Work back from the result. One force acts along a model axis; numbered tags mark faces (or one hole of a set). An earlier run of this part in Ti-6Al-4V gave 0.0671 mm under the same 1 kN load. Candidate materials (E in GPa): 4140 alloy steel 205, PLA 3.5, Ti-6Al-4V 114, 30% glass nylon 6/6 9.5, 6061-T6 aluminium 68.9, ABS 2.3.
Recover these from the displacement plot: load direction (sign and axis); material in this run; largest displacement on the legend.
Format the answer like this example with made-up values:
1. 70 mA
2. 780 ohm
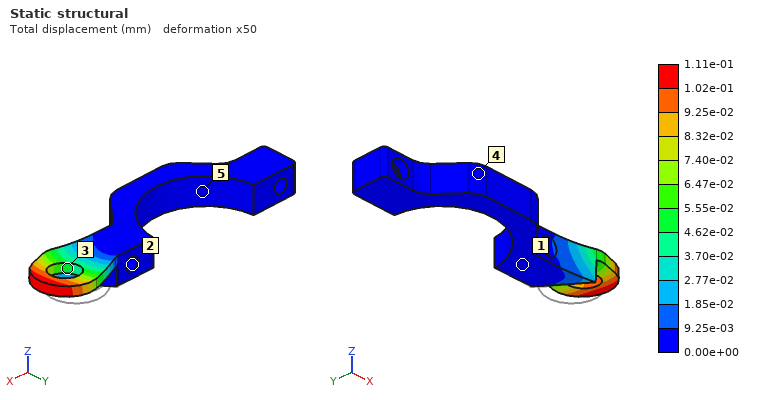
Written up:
1. -Y
2. 6061-T6 aluminium
3. 1.11e-01 mm
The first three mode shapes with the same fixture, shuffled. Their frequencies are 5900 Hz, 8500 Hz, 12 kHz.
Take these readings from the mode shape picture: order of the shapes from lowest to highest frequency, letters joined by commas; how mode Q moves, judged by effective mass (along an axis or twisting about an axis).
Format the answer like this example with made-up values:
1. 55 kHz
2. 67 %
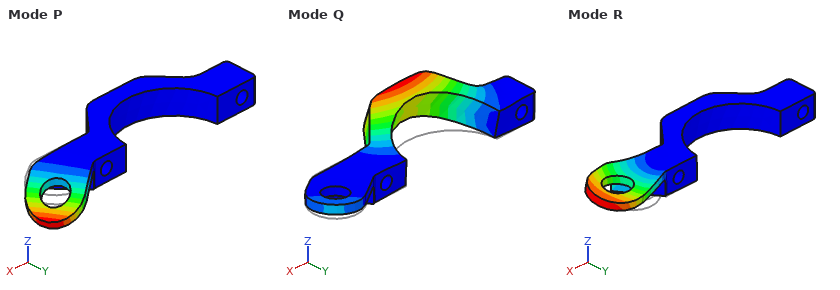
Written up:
1. P, Q, R
2. along Z
